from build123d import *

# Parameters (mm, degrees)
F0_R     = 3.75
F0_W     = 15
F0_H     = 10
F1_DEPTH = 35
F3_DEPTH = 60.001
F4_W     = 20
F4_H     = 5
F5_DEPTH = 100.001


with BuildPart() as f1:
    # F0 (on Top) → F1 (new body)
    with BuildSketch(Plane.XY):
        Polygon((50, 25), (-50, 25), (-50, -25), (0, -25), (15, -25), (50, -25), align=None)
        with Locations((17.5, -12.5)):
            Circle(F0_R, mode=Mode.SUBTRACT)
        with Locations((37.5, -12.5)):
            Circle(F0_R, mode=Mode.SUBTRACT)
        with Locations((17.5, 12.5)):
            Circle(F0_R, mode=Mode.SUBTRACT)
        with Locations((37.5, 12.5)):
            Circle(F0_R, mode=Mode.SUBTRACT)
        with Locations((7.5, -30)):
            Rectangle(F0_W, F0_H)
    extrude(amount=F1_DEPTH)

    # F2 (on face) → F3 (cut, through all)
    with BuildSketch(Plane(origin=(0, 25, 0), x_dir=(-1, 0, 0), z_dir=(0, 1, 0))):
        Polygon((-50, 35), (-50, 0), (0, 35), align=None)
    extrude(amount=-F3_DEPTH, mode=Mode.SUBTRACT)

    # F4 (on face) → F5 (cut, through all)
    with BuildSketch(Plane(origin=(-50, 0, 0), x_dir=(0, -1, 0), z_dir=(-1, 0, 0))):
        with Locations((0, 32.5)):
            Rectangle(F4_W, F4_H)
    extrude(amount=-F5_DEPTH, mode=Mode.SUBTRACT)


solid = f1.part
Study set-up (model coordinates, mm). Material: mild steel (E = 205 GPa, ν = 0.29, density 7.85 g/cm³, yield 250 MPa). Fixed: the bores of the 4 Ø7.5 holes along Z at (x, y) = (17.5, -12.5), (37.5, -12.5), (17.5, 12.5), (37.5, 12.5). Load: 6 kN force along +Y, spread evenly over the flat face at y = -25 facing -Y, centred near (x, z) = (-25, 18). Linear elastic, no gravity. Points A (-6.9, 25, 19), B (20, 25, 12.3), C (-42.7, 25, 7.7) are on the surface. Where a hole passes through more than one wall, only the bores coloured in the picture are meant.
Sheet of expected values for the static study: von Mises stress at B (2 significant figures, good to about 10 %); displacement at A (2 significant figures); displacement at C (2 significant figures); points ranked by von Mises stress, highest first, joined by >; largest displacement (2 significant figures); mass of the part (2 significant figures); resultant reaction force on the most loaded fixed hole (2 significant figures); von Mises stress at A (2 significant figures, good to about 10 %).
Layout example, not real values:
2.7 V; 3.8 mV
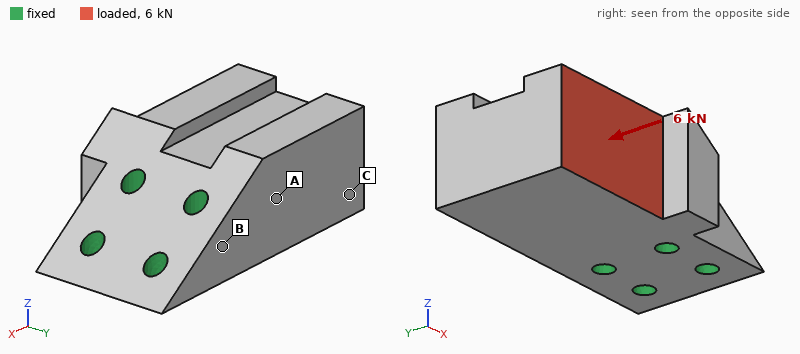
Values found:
14 MPa; 4.0 µm; 8.5 µm; B > A > C; 10 µm; 1.0 kg; 7.9 kN; 7.7 MPa
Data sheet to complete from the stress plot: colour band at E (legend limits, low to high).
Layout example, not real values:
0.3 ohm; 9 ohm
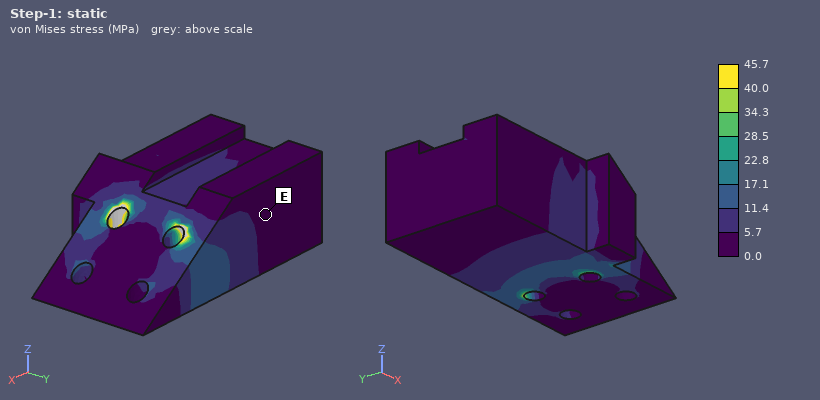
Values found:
0.0 to 5.7 MPa
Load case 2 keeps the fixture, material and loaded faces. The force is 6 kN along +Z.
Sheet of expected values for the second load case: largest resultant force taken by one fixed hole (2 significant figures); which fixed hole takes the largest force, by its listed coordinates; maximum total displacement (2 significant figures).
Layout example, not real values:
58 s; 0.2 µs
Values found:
6.5 kN; (17.5, -12.5); 29 µm
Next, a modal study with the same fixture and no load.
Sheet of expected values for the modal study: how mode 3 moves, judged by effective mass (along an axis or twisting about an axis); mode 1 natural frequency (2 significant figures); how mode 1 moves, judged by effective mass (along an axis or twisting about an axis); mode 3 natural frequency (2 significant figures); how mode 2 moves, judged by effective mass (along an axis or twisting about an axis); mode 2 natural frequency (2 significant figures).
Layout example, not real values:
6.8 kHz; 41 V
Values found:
twisting about X; 3900 Hz; along Z; 9000 Hz; along Y; 5800 Hz
